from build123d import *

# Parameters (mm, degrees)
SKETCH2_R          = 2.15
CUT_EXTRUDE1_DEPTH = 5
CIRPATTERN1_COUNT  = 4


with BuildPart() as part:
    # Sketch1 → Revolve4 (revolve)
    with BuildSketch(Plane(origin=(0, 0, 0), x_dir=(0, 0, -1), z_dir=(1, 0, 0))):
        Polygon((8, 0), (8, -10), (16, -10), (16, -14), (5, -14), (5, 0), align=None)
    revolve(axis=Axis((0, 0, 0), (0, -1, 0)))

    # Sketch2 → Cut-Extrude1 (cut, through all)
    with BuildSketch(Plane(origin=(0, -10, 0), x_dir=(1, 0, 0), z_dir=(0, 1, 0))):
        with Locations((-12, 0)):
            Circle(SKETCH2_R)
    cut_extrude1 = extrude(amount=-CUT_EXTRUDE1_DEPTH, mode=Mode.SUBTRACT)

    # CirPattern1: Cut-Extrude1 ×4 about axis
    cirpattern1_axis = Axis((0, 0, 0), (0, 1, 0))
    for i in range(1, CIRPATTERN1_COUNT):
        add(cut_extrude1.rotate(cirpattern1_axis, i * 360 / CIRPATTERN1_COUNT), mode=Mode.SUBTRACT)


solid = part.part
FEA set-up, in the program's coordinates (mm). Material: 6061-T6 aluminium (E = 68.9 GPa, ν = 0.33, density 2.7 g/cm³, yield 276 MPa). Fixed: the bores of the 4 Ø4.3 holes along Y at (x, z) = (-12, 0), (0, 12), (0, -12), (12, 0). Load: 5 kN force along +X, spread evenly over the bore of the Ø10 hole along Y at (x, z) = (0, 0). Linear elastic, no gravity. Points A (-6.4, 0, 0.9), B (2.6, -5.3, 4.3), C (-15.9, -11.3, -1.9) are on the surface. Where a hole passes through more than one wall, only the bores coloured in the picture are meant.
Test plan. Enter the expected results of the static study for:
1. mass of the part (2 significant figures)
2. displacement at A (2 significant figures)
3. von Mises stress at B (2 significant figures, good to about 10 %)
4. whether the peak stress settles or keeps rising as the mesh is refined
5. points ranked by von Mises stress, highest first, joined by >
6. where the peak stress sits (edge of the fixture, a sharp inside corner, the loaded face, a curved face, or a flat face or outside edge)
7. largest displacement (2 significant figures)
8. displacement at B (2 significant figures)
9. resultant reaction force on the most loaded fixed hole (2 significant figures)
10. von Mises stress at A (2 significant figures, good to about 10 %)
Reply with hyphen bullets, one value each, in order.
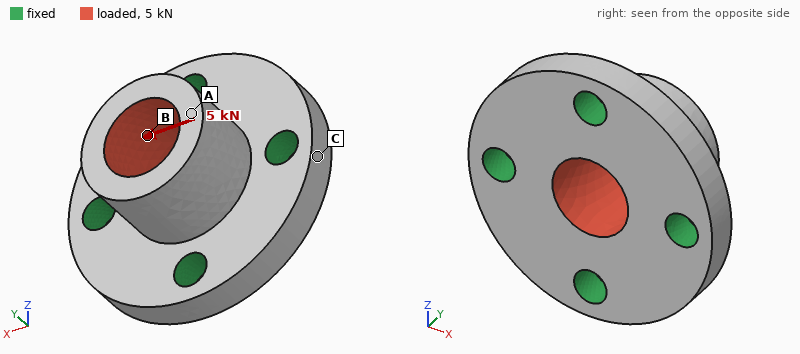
- 11 g
- 26 µm
- 60 MPa
- keeps rising
- B > A > C
- edge of the fixture
- 27 µm
- 15 µm
- 1.9 kN
- 36 MPa
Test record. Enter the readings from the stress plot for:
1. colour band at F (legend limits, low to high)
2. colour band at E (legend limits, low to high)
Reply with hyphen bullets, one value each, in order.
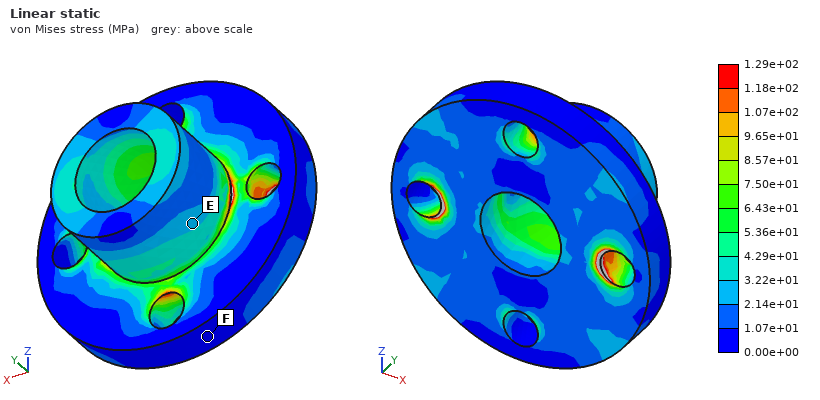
- 0.00e+00 to 1.07e+01 MPa
- 2.14e+01 to 3.22e+01 MPa
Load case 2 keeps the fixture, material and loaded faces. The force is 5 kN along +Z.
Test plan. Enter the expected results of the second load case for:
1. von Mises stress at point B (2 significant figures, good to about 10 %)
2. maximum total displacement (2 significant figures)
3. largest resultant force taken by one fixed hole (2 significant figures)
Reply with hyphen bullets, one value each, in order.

- 45 MPa
- 27 µm
- 1.9 kN
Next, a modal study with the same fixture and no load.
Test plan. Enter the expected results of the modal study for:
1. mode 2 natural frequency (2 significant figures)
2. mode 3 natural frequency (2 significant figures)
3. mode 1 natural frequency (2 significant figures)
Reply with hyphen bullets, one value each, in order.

- 37 kHz
- 49 kHz
- 37 kHz
